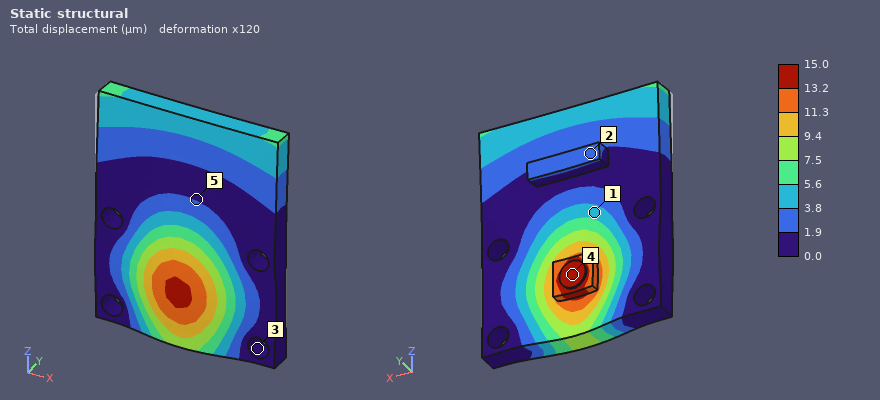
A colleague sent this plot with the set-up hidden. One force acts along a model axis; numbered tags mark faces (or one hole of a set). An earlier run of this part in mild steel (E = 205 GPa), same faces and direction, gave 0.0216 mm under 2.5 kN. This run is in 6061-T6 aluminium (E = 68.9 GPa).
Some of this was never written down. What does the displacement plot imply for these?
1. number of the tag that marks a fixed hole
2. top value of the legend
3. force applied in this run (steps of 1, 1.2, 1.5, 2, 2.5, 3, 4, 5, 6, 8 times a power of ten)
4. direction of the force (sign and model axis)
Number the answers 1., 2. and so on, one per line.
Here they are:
1. 3
2. 15.0 µm
3. 600 N
4. -Y
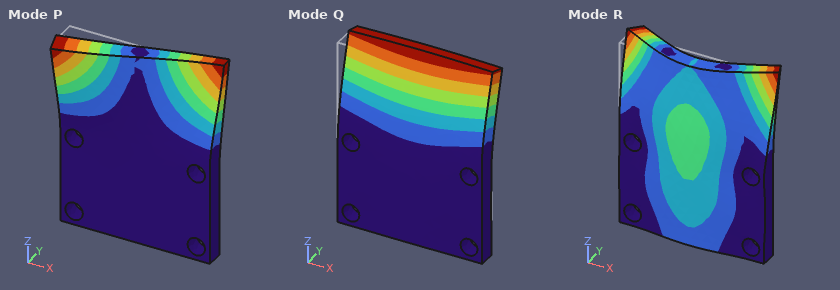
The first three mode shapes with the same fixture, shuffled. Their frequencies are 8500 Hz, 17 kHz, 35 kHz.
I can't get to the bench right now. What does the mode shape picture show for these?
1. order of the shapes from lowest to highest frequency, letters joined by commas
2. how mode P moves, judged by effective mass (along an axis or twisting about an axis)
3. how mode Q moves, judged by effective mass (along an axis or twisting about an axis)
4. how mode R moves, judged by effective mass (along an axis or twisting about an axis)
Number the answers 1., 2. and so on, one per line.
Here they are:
1. Q, P, R
2. twisting about Z
3. along Y
4. along Y
